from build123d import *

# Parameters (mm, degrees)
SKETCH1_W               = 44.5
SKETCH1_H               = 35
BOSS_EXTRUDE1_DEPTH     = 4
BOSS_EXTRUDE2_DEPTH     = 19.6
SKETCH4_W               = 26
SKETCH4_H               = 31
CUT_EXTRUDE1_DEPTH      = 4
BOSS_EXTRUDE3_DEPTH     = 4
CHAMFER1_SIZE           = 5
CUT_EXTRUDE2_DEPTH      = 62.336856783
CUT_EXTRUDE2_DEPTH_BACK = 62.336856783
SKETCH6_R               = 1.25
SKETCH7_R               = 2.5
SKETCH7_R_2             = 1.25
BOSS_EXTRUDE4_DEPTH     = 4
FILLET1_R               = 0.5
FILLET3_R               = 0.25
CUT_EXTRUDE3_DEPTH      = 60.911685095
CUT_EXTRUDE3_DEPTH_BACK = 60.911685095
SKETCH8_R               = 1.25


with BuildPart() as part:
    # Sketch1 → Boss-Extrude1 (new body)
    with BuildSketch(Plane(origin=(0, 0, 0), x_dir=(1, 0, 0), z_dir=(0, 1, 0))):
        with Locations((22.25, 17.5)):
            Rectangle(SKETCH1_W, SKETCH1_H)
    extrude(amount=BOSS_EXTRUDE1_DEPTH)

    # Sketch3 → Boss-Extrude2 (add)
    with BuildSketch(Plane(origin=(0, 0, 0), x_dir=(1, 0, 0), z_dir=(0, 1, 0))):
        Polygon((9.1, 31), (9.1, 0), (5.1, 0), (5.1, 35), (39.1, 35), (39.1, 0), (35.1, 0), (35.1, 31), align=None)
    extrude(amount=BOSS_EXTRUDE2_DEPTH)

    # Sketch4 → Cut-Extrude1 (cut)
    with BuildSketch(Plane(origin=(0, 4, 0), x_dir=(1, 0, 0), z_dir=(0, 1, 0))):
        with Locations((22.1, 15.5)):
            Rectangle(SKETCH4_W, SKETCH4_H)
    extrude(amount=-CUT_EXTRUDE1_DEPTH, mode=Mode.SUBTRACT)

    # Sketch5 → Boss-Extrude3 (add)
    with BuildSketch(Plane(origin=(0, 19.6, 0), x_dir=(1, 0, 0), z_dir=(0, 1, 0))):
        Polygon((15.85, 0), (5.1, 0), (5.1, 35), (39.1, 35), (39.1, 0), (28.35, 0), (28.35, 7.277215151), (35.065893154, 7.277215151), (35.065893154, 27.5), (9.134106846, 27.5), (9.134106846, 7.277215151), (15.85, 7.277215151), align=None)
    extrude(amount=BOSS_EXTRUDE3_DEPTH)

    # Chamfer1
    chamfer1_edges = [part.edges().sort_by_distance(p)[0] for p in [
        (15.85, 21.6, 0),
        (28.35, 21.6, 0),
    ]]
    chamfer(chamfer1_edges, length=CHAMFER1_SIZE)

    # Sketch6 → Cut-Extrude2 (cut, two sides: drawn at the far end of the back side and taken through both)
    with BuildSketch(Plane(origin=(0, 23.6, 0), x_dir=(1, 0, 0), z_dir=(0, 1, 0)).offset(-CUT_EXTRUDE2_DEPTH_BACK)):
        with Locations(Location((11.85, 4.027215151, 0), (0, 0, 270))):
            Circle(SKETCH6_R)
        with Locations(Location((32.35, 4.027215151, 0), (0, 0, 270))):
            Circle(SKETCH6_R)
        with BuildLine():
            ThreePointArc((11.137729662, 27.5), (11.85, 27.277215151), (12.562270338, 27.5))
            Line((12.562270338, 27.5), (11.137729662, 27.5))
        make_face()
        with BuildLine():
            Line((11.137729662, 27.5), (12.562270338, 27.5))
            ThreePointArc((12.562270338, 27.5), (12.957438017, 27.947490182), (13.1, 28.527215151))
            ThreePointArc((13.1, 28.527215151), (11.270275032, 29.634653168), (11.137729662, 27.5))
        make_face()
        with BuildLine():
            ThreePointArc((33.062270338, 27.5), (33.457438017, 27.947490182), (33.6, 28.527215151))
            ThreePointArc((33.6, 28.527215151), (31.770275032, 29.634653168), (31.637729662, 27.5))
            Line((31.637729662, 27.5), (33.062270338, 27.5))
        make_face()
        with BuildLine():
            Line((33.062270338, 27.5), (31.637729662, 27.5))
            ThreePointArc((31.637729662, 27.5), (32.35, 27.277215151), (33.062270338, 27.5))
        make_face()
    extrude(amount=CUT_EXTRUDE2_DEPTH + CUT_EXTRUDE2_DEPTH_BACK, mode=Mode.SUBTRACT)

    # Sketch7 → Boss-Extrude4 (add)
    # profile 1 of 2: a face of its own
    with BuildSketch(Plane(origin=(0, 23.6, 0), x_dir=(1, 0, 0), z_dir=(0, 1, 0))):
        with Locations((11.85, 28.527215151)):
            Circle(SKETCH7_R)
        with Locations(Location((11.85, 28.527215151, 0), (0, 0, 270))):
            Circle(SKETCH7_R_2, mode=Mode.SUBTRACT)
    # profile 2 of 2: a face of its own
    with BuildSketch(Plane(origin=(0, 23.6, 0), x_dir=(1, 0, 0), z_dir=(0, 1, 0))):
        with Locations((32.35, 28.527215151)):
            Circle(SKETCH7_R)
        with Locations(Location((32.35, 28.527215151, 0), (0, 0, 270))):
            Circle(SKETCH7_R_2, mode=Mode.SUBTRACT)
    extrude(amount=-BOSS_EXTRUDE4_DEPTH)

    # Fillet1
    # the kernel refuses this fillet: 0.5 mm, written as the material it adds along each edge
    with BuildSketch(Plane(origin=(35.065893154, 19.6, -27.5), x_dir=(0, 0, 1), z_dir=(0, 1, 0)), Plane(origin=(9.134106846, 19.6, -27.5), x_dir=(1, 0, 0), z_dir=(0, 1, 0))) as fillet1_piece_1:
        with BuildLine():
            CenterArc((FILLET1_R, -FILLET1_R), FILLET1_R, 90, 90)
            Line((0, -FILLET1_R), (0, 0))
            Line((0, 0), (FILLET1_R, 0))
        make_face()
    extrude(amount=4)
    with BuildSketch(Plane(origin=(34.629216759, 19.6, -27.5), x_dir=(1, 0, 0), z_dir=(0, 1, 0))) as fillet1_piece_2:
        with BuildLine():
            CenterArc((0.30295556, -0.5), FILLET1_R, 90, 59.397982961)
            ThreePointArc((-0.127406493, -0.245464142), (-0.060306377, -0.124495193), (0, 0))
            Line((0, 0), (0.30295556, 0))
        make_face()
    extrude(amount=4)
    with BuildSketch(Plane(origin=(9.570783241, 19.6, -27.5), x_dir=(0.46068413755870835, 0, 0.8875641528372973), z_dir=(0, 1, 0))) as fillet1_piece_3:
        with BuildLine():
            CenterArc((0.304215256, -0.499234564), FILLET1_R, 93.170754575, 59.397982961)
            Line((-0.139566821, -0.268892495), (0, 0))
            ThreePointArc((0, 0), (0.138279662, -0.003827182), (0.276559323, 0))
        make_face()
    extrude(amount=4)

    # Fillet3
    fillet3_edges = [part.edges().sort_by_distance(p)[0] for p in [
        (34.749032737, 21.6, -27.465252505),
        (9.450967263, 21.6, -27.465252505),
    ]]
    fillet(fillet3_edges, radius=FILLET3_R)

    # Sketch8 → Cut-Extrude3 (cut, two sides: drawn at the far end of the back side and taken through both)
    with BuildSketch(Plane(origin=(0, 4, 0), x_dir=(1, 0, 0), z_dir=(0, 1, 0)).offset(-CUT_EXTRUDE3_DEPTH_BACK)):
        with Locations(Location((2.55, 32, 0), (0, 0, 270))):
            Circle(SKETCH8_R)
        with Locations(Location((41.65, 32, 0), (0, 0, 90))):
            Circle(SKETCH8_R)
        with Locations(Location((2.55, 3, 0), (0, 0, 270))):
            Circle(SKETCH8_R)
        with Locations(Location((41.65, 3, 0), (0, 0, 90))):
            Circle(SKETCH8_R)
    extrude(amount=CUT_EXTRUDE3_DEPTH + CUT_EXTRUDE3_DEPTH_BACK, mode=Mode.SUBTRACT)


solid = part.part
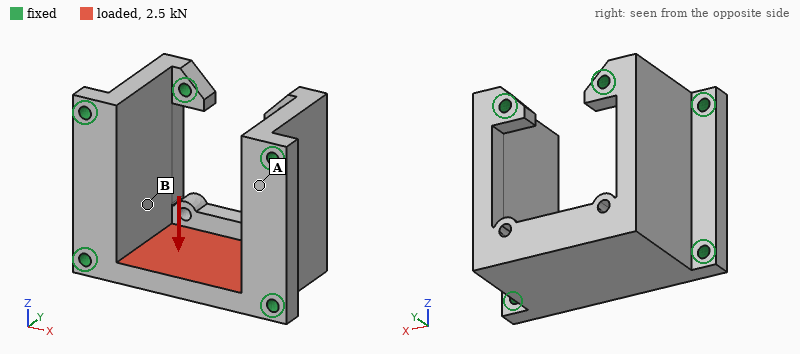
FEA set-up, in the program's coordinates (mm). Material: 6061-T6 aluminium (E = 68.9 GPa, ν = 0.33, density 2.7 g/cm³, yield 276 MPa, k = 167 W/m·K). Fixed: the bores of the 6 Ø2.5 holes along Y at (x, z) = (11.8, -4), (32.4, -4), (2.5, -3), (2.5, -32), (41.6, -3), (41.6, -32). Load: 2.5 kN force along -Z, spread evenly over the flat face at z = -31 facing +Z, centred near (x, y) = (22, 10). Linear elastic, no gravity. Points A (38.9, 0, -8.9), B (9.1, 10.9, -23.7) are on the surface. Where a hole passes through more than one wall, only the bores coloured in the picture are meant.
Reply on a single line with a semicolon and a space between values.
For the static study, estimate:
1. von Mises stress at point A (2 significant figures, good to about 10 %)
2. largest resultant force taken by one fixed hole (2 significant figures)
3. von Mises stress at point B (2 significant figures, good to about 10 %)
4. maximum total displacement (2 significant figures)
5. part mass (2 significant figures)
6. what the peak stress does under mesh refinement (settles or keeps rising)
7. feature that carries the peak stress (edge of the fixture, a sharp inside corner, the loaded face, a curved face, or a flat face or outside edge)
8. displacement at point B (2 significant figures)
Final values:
14 MPa; 660 N; 30 MPa; 50 µm; 30 g; keeps rising; edge of the fixture; 11 µm
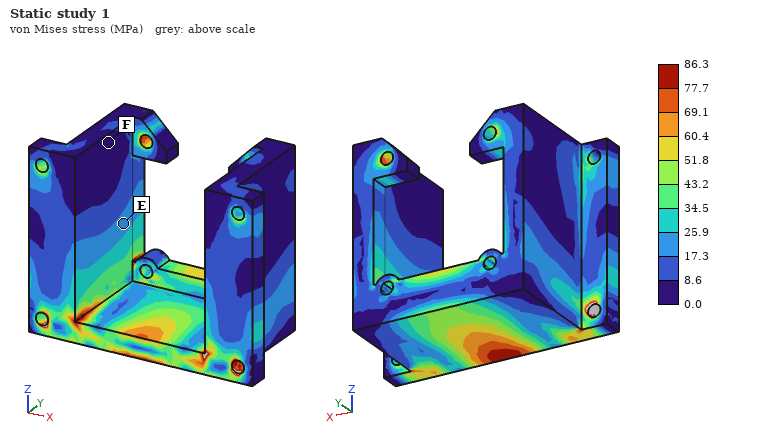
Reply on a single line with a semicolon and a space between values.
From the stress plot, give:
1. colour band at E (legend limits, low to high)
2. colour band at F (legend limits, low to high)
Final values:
17.3 to 25.9 MPa; 0.0 to 8.6 MPa
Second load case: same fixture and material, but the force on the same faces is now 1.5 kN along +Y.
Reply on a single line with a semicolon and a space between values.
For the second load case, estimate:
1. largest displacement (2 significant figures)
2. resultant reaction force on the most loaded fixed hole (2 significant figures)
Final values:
13 µm; 710 N
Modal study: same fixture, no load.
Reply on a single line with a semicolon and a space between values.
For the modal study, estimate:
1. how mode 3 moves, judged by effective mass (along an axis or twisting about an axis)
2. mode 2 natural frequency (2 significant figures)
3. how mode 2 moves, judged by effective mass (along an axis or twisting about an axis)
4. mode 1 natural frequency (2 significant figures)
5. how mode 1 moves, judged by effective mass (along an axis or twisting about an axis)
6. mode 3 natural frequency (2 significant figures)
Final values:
along Y; 18 kHz; along X; 14 kHz; along Z; 19 kHz
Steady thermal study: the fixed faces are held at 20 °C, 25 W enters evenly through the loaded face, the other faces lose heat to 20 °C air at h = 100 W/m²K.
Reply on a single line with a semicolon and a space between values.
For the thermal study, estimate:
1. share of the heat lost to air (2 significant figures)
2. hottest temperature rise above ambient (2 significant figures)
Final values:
12 %; 15 K
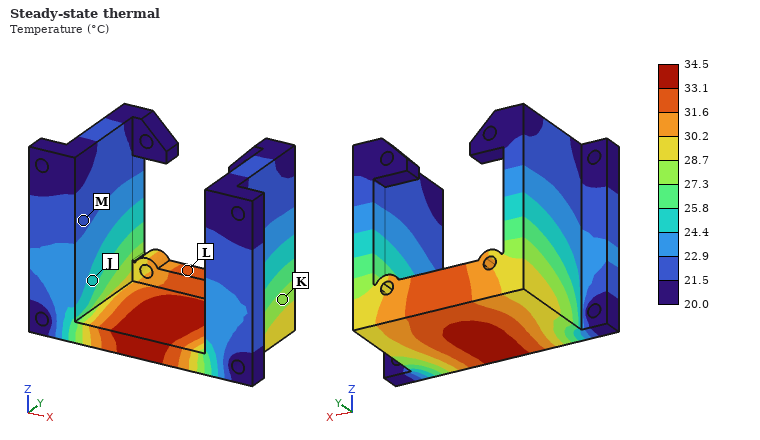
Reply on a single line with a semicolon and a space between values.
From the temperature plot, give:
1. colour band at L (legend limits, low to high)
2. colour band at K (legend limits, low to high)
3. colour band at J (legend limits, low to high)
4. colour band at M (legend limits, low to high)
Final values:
31.6 to 33.1 °C; 27.3 to 28.7 °C; 24.4 to 25.8 °C; 21.5 to 22.9 °C
